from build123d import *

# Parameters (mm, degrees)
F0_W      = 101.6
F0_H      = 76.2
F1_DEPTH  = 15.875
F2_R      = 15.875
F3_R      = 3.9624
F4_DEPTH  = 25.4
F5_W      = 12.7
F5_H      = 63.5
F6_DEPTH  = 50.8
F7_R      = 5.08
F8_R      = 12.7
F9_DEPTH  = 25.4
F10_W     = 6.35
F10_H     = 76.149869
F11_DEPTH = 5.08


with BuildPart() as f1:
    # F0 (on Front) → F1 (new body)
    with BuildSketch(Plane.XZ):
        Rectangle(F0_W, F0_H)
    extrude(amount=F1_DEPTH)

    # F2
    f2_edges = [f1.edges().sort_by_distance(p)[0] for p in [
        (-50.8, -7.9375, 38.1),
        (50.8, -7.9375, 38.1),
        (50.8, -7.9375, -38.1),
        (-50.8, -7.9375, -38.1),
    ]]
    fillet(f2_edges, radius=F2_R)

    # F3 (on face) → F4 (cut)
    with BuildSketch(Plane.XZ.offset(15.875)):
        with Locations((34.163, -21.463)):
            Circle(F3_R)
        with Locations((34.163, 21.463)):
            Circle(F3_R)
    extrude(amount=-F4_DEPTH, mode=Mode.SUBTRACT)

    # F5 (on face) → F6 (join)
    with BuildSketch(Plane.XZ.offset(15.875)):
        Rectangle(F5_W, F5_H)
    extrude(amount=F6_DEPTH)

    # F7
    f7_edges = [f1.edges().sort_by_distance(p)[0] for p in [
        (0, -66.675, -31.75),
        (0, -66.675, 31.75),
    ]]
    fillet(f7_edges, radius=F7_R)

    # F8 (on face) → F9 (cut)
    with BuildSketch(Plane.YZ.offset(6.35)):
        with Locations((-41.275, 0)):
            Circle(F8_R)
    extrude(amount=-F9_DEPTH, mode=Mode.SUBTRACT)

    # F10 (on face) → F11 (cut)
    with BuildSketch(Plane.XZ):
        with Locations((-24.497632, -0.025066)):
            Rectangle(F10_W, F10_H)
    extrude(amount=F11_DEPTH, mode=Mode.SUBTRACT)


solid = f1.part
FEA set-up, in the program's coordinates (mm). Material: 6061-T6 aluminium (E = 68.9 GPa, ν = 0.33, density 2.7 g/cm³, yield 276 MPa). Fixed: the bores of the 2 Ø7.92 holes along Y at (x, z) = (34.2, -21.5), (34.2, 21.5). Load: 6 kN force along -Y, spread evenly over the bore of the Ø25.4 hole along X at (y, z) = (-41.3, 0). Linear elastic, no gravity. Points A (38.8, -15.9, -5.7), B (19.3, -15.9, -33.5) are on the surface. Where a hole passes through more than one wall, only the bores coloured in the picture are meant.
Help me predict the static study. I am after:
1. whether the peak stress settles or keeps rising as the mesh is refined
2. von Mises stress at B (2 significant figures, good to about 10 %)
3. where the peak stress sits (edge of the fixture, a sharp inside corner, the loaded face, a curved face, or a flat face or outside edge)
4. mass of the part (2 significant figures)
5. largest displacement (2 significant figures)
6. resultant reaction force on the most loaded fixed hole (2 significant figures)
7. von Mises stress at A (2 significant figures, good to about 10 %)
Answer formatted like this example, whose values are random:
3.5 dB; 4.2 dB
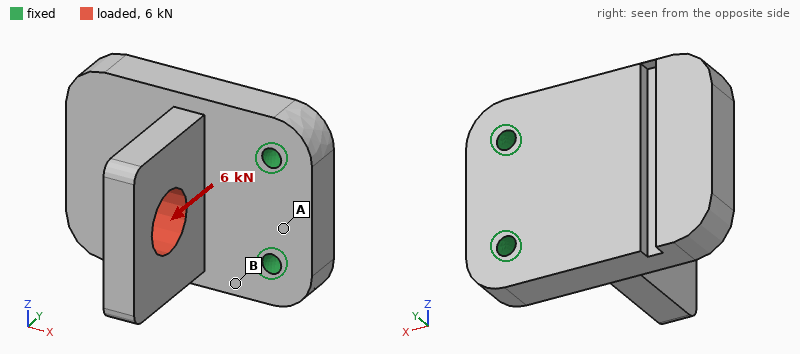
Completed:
keeps rising; 34 MPa; edge of the fixture; 400 g; 0.18 mm; 3.0 kN; 15 MPa
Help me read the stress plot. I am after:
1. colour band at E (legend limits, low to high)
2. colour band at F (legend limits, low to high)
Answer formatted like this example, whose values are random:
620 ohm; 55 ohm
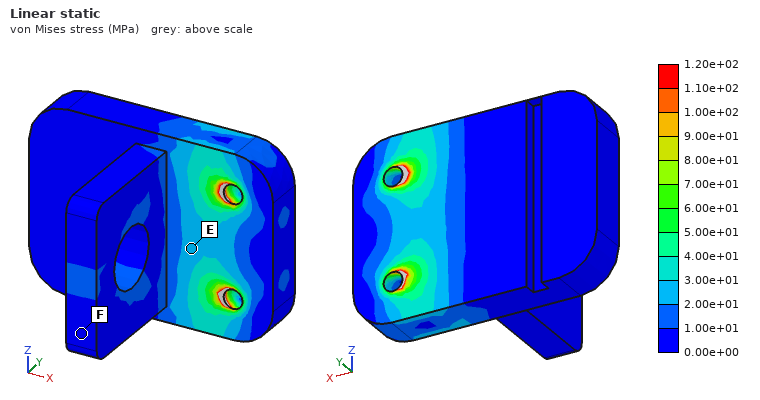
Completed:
2.00e+01 to 3.00e+01 MPa; 0.00e+00 to 1.00e+01 MPa
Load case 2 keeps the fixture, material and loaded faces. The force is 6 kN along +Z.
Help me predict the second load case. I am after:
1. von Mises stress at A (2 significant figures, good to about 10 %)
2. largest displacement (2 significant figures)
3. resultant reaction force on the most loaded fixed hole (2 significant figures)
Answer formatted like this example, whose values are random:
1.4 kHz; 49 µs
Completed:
9.8 MPa; 0.12 mm; 6.3 kN
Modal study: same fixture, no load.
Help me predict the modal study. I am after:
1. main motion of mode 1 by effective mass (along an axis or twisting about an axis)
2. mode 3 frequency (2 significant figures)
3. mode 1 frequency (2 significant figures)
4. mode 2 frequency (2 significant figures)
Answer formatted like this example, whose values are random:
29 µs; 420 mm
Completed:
along Y; 3600 Hz; 1500 Hz; 3400 Hz
